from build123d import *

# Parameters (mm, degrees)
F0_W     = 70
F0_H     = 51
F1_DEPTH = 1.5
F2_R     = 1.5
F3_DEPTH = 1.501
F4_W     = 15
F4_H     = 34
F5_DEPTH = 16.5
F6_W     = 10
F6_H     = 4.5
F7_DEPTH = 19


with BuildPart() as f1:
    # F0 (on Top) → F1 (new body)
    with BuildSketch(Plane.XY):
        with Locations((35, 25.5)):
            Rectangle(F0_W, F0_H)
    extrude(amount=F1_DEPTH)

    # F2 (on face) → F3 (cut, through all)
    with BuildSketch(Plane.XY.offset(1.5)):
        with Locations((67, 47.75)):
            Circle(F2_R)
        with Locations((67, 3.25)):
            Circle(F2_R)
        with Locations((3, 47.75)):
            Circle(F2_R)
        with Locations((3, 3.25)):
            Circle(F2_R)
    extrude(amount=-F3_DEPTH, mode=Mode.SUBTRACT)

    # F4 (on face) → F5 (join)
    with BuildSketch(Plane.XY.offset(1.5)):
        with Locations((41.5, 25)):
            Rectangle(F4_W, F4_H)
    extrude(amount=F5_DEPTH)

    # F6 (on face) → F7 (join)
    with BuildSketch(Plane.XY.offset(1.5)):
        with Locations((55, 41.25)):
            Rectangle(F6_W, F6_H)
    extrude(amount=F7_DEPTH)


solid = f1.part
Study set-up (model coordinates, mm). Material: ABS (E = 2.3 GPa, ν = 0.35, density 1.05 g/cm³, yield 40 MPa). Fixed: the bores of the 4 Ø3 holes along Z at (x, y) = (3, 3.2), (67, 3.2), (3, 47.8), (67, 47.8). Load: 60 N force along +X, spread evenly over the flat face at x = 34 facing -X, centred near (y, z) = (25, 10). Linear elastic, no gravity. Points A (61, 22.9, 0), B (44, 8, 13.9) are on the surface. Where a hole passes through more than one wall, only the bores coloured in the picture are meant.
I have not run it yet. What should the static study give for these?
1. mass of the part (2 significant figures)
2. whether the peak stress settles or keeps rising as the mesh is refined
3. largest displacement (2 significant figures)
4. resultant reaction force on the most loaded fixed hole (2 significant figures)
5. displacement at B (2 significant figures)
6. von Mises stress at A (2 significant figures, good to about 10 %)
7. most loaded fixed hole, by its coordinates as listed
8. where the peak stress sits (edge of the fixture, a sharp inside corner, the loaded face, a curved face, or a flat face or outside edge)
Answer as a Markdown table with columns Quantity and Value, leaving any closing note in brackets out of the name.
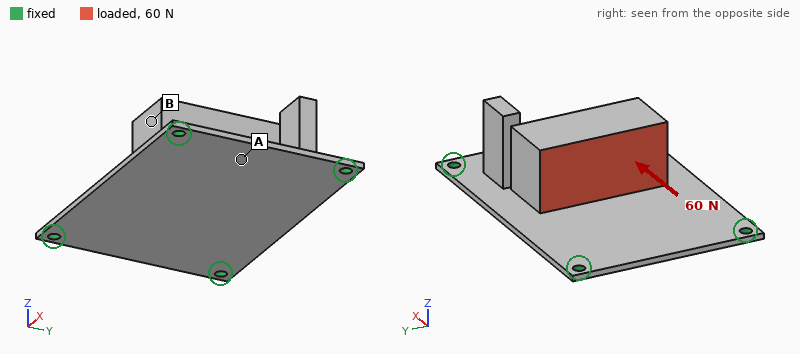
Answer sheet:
| Quantity | Value |
|---|---|
| mass of the part | 15 g |
| whether the peak stress settles or keeps rising as the mesh is refined | keeps rising |
| largest displacement | 0.84 mm |
| resultant reaction force on the most loaded fixed hole | 20 N |
| displacement at B | 0.51 mm |
| von Mises stress at A | 2.3 MPa |
| most loaded fixed hole, by its coordinates as listed | (67, 47.8) |
| where the peak stress sits | edge of the fixture |
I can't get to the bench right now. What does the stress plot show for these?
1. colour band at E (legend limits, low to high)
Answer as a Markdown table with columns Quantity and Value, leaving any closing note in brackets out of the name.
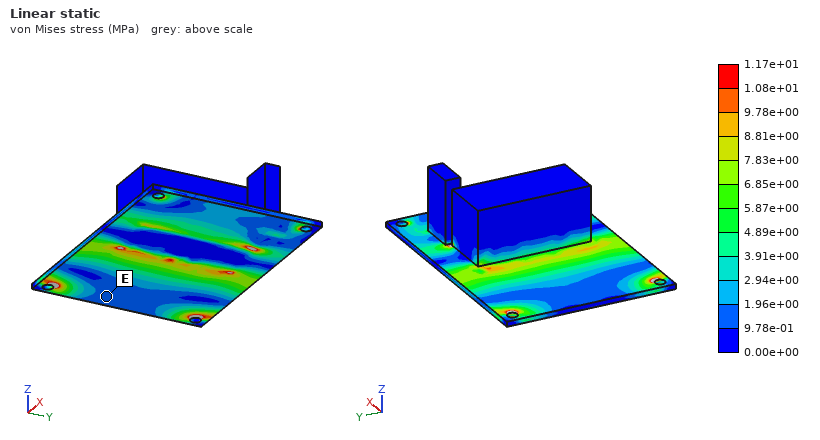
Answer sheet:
| Quantity | Value |
|---|---|
| colour band at E | 9.78e-01 to 1.96e+00 MPa |
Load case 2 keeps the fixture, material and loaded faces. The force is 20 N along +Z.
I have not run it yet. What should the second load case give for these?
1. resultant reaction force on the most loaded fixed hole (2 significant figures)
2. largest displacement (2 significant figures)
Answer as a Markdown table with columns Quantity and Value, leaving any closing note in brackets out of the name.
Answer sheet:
| Quantity | Value |
|---|---|
| resultant reaction force on the most loaded fixed hole | 5.8 N |
| largest displacement | 0.90 mm |
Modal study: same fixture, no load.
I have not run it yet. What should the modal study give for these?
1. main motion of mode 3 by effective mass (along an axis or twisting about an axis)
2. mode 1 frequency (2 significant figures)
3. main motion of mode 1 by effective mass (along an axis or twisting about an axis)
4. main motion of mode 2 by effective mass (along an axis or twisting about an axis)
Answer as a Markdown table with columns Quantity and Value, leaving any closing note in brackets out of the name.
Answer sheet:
| Quantity | Value |
|---|---|
| main motion of mode 3 by effective mass | along X |
| mode 1 frequency | 260 Hz |
| main motion of mode 1 by effective mass | along Z |
| main motion of mode 2 by effective mass | along Y |
